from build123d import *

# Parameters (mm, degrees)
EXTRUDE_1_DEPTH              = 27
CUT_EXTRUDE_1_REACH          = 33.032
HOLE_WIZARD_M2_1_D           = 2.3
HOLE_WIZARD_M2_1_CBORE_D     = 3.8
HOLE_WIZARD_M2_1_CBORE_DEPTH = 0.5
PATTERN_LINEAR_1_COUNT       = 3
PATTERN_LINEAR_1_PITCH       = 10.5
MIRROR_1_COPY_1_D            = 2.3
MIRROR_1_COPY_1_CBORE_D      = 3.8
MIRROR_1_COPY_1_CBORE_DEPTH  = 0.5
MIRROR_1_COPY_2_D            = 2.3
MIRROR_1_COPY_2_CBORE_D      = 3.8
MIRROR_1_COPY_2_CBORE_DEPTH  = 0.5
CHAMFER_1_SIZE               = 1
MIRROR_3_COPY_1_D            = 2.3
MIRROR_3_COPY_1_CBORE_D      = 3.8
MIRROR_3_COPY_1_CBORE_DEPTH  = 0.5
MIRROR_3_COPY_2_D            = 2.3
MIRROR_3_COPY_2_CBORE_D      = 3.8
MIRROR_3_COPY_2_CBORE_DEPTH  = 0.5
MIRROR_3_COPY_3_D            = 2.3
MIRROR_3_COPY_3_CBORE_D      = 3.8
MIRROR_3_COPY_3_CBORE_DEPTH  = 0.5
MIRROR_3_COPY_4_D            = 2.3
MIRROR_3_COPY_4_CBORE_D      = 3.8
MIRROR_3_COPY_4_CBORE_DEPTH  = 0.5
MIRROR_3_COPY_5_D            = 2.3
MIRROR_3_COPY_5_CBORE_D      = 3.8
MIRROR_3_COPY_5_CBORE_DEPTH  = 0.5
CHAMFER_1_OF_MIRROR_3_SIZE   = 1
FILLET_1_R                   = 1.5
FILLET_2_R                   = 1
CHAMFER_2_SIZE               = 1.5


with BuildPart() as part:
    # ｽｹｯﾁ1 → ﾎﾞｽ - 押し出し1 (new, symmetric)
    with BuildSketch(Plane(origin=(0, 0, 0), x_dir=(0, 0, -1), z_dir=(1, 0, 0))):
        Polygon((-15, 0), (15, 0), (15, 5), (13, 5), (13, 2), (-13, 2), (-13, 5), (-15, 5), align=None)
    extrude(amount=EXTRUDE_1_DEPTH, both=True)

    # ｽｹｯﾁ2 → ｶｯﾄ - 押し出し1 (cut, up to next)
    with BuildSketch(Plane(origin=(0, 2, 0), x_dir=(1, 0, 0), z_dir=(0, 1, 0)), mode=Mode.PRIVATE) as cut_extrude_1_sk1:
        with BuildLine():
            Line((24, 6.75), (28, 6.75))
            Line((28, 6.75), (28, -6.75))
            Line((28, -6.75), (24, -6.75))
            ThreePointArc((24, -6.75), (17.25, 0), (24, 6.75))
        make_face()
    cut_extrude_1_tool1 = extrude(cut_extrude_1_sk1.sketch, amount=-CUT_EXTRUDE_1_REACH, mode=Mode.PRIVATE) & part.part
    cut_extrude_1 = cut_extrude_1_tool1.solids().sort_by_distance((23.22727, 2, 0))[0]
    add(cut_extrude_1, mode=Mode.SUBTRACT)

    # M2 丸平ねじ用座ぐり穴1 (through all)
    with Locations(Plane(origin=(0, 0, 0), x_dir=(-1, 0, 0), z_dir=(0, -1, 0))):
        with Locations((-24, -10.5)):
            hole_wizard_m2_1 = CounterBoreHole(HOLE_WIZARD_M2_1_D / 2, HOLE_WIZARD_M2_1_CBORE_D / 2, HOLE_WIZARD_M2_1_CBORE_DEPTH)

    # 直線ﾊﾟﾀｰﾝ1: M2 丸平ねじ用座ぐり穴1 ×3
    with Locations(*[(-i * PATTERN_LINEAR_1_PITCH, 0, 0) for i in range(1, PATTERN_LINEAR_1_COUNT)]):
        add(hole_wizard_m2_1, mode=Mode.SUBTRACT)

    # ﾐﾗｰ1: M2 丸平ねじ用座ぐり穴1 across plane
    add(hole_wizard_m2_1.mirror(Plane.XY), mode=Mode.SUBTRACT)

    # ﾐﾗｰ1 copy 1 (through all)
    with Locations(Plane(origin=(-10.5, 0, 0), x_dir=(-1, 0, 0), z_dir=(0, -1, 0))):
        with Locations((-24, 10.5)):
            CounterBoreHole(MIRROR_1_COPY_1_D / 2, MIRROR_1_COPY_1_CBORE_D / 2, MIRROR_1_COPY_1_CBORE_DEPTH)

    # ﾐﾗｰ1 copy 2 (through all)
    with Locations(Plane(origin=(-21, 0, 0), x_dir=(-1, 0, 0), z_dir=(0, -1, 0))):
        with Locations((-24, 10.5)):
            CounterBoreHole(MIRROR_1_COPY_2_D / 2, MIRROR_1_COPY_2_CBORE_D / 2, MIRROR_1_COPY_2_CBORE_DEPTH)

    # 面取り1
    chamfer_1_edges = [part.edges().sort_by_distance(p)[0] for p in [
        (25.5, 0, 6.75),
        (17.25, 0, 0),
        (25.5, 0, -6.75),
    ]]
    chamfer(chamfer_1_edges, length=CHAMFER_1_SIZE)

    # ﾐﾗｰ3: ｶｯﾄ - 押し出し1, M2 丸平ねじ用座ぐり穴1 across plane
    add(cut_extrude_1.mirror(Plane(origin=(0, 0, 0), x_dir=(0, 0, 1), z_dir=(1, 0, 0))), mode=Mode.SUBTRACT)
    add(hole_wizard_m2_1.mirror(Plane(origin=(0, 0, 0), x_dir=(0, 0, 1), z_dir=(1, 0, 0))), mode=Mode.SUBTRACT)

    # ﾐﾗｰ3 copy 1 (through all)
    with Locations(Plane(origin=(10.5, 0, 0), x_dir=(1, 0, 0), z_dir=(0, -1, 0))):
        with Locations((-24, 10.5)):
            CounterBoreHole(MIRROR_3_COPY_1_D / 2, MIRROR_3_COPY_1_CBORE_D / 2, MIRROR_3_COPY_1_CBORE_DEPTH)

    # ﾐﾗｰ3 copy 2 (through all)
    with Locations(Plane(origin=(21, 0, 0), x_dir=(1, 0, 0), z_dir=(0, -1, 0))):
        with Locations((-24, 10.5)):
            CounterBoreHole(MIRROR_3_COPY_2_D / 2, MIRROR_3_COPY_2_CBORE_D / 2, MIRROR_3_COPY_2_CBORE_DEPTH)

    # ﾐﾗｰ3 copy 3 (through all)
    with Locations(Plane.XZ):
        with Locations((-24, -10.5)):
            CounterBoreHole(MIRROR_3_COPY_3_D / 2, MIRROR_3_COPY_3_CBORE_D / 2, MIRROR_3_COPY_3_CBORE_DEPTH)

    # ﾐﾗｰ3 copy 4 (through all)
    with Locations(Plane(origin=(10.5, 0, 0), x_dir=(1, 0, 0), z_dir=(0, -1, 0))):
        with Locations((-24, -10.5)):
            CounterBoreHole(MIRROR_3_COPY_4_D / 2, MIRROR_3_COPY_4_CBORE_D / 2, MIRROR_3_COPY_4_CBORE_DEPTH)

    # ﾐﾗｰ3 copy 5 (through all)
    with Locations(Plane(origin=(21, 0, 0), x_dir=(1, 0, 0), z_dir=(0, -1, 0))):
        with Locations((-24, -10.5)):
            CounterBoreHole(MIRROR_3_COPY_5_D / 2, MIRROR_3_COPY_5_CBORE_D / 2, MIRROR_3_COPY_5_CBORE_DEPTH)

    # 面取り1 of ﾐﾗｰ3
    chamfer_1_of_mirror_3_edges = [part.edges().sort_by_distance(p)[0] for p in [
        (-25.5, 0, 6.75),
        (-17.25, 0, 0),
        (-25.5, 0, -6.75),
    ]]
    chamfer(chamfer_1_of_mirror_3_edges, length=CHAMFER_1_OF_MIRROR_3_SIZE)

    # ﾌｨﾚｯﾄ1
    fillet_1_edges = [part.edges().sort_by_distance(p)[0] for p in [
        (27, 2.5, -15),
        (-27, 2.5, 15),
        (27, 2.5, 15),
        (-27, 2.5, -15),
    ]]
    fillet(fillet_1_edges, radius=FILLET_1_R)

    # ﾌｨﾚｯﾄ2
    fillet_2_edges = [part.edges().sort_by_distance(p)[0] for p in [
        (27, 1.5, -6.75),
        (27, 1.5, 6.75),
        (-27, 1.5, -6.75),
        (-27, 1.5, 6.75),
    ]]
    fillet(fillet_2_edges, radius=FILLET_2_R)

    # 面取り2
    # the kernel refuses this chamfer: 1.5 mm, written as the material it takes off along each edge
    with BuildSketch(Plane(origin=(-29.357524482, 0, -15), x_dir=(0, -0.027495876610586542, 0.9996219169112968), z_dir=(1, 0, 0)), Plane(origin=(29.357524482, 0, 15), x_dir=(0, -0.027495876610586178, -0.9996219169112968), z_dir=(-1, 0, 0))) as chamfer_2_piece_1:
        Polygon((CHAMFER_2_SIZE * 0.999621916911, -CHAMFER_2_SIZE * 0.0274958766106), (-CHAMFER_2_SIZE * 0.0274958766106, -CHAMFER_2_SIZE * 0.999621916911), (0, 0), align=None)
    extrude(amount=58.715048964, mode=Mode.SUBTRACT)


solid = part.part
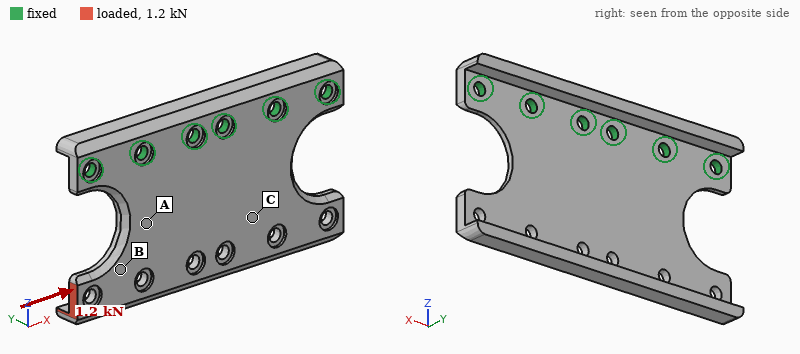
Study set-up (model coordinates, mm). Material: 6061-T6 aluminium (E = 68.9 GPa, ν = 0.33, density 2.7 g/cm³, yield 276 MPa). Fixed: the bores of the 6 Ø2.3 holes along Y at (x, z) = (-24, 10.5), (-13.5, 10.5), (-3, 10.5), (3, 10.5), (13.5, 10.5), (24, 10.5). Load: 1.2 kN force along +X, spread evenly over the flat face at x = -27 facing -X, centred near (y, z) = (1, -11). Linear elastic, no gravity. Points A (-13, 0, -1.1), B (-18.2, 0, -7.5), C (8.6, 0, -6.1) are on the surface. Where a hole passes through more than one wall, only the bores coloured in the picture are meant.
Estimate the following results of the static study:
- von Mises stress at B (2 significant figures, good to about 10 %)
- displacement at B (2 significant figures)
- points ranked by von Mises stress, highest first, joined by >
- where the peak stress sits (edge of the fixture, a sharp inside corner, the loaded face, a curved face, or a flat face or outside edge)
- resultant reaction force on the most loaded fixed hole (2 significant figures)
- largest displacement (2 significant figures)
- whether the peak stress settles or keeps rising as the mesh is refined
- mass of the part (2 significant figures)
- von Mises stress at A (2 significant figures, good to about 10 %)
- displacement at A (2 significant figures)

74 MPa
39 µm
B > A > C
a sharp inside corner
610 N
83 µm
keeps rising
8.5 g
40 MPa
17 µm
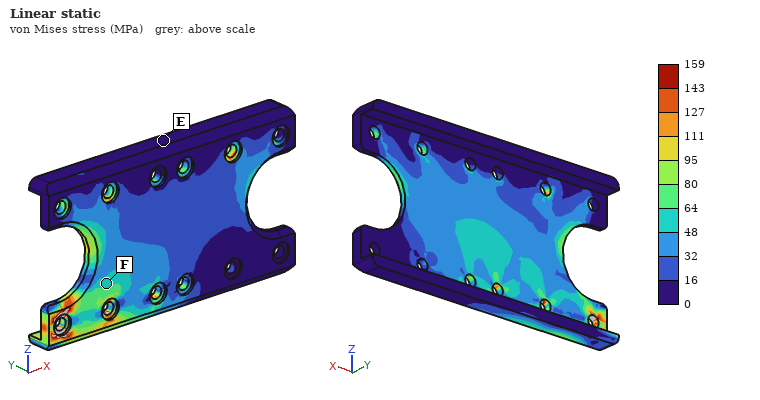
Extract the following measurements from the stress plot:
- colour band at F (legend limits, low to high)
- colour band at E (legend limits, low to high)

48 to 64 MPa
0 to 16 MPa
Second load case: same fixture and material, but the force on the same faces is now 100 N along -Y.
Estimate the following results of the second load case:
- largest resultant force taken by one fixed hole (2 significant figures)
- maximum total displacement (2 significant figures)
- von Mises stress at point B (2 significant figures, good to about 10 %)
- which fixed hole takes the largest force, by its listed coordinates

130 N
0.71 mm
97 MPa
(-13.5, 10.5)
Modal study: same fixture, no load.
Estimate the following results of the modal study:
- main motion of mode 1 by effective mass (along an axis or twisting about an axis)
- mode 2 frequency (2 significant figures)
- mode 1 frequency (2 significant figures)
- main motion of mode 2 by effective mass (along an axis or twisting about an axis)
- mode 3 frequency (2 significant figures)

along Y
2600 Hz
1900 Hz
twisting about Z
8300 Hz
